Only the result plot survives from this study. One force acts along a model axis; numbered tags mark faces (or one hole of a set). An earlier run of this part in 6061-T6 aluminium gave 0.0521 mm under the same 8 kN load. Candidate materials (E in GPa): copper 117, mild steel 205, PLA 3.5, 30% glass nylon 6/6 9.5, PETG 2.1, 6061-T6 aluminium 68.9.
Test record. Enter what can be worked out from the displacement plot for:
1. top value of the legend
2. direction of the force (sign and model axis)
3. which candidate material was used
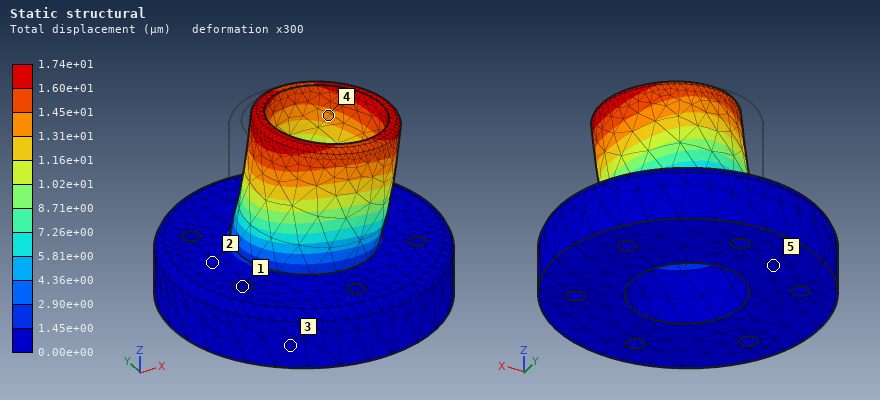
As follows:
1.74e+01 µm
+X
mild steel
